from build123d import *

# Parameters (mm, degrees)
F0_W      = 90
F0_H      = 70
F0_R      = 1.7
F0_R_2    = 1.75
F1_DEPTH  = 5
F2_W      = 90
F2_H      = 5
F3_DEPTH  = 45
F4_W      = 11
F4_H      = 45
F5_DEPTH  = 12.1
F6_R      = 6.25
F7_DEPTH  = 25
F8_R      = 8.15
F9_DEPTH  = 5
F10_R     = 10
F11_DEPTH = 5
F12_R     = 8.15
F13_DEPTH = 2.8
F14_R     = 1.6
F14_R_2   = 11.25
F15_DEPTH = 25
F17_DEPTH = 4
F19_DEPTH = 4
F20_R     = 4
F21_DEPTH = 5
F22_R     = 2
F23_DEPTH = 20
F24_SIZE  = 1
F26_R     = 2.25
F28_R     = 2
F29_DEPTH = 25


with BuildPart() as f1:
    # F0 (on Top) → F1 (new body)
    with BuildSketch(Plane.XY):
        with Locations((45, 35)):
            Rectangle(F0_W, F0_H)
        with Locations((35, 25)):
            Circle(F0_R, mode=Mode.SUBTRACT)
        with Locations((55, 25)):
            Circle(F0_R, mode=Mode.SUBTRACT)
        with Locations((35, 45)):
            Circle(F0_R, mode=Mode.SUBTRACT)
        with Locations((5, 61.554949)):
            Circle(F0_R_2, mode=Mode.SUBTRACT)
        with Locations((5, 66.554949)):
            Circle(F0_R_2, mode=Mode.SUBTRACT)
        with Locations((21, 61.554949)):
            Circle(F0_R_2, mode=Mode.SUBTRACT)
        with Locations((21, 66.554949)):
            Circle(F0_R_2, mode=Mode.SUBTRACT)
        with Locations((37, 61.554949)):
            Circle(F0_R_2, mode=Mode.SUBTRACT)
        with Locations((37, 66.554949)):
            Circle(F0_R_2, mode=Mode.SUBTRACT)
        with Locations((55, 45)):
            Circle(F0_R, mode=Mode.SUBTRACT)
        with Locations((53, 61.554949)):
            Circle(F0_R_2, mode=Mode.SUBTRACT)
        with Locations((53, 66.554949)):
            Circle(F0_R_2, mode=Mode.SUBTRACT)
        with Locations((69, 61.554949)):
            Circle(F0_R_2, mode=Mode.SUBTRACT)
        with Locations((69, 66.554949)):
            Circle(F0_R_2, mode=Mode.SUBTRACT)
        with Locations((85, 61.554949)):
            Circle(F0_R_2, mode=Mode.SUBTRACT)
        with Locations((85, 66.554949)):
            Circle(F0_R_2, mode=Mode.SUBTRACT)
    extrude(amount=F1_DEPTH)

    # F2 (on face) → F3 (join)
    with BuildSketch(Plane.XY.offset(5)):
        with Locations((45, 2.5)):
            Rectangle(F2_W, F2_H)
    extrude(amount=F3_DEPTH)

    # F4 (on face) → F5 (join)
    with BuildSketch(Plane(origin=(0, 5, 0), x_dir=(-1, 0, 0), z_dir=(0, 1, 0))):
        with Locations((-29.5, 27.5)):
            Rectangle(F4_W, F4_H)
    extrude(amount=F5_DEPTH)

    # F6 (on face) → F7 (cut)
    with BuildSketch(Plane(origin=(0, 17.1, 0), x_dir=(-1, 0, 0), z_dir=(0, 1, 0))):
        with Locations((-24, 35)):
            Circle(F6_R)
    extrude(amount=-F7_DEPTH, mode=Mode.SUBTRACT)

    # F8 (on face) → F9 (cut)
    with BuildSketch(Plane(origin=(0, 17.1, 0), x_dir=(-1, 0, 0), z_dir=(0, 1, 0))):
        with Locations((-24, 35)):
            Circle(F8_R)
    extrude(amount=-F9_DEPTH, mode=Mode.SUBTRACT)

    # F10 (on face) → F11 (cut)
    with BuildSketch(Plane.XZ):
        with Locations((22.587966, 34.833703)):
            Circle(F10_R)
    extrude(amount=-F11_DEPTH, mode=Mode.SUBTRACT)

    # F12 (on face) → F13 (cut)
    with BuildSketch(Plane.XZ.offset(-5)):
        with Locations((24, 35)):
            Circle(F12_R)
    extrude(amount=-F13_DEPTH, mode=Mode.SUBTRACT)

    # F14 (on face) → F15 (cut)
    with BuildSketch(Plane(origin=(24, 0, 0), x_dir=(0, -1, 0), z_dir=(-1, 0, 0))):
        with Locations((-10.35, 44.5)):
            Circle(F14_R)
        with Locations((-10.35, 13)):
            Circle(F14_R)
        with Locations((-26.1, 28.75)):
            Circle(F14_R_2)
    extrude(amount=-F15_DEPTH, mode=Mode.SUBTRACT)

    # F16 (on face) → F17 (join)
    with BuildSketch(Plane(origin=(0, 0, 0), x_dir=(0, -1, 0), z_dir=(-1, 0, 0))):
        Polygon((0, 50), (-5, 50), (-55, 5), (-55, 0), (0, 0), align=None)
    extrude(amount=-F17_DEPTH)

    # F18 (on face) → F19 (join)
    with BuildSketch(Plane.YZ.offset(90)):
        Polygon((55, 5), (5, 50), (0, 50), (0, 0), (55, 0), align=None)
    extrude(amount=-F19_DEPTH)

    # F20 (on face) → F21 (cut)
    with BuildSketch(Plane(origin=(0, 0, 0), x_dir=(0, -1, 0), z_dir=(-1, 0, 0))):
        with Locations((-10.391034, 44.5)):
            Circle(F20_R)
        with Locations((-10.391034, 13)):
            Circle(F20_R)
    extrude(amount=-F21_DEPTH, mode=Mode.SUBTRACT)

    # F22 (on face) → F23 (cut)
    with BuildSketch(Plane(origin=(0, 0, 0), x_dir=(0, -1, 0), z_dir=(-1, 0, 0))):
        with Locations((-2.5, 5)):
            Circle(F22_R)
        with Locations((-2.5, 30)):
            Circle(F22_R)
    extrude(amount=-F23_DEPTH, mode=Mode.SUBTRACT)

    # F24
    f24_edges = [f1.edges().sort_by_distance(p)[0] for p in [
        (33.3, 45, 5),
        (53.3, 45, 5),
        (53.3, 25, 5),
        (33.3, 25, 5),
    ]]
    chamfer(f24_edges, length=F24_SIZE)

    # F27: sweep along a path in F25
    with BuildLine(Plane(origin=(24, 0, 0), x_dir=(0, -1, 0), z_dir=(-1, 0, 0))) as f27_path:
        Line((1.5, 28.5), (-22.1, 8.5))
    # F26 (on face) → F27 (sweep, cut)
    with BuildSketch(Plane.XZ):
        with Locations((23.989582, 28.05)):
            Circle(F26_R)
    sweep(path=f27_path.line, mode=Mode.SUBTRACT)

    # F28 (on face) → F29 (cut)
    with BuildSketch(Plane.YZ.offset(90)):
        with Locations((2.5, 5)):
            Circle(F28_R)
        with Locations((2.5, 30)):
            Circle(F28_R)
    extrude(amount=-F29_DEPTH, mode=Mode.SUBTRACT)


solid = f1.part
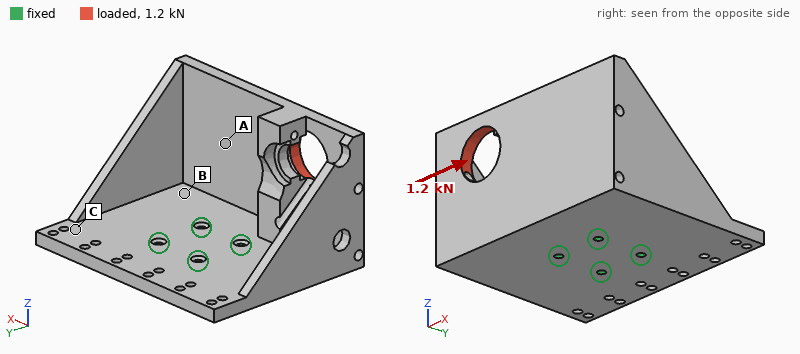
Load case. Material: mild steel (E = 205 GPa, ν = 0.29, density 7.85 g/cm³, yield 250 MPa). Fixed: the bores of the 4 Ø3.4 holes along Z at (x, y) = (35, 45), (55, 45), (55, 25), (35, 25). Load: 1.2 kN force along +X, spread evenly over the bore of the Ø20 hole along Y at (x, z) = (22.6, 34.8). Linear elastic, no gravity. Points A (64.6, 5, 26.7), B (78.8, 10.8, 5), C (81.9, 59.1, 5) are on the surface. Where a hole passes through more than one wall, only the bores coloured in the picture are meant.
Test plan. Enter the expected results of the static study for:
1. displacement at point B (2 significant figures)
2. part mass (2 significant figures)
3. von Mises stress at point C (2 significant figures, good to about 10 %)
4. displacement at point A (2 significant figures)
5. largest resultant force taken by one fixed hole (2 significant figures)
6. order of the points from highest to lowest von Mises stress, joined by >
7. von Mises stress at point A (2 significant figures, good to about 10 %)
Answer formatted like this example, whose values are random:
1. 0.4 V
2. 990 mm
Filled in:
1. 0.041 mm
2. 480 g
3. 15 MPa
4. 0.047 mm
5. 1.6 kN
6. A > C > B
7. 26 MPa
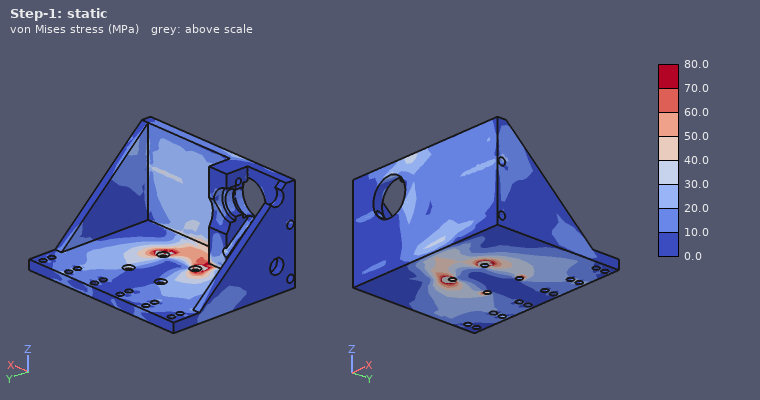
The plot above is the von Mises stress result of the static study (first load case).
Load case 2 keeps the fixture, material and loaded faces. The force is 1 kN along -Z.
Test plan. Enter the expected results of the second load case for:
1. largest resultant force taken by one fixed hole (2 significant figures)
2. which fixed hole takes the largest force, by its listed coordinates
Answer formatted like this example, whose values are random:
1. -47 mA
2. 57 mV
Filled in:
1. 1.6 kN
2. (35, 25)
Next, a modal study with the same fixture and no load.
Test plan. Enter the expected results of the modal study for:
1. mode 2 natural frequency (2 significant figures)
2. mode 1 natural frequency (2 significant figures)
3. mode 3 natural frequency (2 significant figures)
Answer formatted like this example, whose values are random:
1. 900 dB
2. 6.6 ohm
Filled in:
1. 1400 Hz
2. 1300 Hz
3. 2600 Hz
